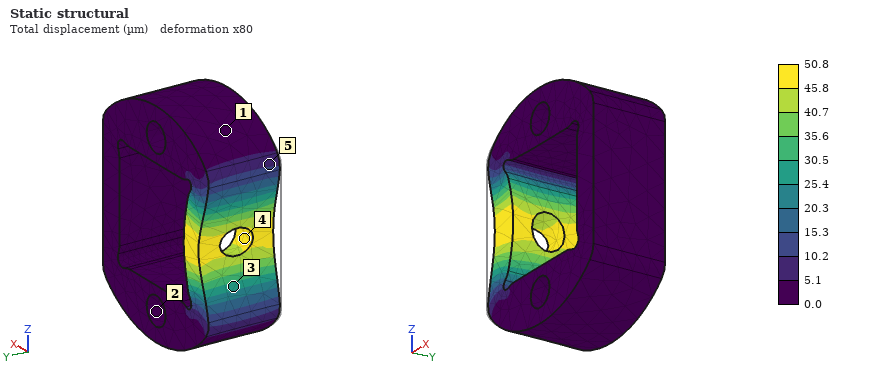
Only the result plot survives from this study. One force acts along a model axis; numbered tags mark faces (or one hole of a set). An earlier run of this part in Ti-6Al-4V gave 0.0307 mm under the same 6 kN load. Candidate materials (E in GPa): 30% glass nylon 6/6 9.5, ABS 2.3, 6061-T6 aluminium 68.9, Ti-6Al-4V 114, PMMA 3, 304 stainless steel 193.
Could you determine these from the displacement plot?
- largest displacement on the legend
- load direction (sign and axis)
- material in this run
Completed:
50.8 µm
+X
6061-T6 aluminium
